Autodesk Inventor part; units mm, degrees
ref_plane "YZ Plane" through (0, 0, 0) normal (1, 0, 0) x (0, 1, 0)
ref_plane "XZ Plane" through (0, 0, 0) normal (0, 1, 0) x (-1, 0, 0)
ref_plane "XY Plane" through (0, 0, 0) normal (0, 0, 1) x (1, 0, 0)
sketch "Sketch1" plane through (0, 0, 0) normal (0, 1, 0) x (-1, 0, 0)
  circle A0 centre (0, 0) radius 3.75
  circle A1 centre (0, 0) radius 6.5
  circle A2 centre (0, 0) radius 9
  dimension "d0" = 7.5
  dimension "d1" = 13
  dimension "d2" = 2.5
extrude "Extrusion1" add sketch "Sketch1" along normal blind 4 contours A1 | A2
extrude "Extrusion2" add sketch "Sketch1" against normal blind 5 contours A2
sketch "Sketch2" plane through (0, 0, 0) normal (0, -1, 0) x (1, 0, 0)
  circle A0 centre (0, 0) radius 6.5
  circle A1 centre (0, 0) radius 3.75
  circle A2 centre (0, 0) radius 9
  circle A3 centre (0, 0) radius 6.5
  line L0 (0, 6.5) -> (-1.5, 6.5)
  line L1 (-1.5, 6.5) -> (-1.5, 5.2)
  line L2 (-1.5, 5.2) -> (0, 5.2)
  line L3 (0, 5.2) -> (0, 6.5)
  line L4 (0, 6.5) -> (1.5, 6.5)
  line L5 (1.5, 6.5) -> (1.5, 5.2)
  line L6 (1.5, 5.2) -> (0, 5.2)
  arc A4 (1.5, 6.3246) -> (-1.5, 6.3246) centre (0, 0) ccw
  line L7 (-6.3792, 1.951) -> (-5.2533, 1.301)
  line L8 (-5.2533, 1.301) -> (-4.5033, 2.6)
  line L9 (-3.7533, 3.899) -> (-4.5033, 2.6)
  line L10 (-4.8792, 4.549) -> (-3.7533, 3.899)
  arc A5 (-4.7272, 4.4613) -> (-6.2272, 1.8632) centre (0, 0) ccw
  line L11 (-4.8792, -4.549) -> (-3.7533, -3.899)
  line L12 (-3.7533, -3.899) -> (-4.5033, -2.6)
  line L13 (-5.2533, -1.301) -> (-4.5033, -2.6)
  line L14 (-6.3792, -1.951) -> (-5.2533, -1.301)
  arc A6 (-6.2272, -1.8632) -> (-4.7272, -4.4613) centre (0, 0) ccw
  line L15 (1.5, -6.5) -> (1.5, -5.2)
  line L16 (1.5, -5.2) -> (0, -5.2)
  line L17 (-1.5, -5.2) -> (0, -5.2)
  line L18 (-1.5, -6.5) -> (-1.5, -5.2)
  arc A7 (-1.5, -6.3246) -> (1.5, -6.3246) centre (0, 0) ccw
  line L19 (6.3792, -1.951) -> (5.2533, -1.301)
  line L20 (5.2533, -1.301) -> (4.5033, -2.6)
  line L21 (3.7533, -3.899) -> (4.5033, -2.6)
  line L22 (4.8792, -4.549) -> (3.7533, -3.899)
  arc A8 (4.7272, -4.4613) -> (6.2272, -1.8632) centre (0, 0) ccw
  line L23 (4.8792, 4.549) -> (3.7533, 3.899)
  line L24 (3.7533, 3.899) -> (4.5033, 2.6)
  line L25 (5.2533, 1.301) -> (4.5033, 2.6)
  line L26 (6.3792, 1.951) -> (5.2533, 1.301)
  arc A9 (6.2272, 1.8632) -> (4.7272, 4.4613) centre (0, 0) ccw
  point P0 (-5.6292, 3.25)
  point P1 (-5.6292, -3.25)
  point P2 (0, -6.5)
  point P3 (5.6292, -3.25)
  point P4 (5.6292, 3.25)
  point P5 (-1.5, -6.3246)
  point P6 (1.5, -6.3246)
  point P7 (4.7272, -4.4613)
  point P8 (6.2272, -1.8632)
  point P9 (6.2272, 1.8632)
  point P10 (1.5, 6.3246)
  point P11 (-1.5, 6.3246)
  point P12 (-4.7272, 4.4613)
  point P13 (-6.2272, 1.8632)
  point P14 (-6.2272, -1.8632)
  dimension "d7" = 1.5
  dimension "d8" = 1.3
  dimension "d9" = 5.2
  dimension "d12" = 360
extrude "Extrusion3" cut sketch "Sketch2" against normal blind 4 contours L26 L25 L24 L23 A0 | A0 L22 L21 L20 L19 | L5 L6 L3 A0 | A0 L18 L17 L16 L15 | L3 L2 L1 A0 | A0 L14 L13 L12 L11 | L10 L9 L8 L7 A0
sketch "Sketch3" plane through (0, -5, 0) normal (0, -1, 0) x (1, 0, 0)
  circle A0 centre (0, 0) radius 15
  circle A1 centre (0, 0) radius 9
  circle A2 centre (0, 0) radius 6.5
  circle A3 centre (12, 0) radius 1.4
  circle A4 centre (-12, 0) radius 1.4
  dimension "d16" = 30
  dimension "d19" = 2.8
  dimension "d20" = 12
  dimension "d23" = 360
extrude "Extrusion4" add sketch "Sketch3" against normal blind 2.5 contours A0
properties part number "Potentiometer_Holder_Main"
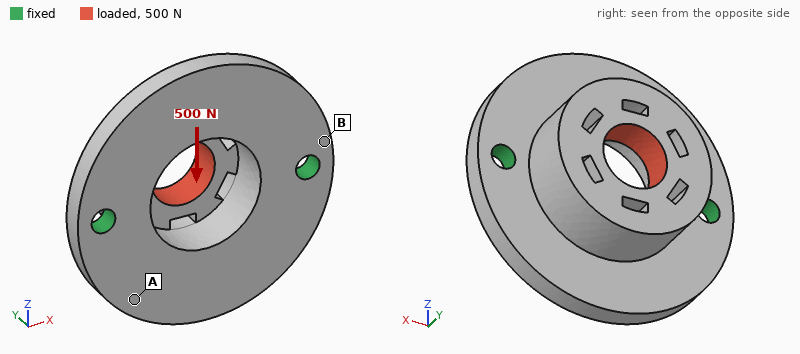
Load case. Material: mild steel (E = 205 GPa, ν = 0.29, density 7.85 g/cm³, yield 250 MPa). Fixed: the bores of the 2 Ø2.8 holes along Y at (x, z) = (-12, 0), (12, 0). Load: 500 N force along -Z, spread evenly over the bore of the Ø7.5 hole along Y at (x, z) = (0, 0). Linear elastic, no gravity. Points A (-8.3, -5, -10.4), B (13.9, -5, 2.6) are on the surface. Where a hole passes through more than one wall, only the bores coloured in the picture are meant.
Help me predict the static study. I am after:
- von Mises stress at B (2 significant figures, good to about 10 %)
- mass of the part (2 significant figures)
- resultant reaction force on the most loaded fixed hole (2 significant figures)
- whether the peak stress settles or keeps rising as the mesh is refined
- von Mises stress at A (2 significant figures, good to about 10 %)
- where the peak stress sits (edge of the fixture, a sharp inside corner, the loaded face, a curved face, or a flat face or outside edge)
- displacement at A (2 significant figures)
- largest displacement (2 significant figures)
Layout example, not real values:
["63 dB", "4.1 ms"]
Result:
["46 MPa", "19 g", "250 N", "keeps rising", "16 MPa", "edge of the fixture", "9.1 µm", "15 µm"]
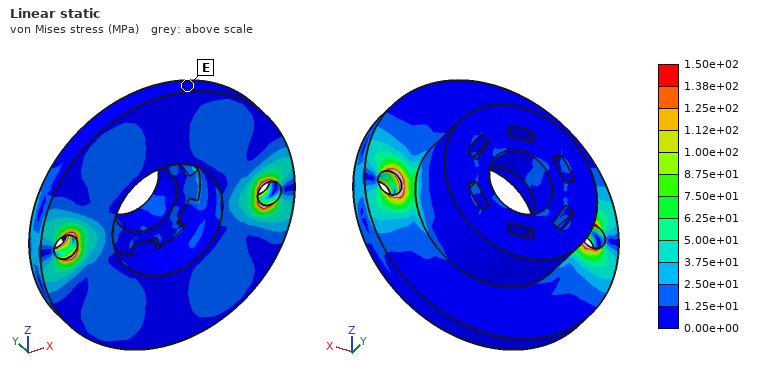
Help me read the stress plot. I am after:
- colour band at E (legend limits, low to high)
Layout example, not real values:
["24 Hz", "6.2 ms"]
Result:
["0.00e+00 to 1.25e+01 MPa"]
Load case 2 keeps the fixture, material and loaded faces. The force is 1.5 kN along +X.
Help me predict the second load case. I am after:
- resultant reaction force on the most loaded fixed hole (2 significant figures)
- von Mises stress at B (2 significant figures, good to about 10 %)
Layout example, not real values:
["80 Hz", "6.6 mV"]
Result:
["860 N", "29 MPa"]
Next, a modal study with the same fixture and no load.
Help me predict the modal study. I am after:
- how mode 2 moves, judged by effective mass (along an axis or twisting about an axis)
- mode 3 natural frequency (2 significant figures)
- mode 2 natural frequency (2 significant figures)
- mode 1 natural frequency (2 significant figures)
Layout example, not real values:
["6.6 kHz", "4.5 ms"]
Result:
["along Y", "30 kHz", "18 kHz", "8000 Hz"]
